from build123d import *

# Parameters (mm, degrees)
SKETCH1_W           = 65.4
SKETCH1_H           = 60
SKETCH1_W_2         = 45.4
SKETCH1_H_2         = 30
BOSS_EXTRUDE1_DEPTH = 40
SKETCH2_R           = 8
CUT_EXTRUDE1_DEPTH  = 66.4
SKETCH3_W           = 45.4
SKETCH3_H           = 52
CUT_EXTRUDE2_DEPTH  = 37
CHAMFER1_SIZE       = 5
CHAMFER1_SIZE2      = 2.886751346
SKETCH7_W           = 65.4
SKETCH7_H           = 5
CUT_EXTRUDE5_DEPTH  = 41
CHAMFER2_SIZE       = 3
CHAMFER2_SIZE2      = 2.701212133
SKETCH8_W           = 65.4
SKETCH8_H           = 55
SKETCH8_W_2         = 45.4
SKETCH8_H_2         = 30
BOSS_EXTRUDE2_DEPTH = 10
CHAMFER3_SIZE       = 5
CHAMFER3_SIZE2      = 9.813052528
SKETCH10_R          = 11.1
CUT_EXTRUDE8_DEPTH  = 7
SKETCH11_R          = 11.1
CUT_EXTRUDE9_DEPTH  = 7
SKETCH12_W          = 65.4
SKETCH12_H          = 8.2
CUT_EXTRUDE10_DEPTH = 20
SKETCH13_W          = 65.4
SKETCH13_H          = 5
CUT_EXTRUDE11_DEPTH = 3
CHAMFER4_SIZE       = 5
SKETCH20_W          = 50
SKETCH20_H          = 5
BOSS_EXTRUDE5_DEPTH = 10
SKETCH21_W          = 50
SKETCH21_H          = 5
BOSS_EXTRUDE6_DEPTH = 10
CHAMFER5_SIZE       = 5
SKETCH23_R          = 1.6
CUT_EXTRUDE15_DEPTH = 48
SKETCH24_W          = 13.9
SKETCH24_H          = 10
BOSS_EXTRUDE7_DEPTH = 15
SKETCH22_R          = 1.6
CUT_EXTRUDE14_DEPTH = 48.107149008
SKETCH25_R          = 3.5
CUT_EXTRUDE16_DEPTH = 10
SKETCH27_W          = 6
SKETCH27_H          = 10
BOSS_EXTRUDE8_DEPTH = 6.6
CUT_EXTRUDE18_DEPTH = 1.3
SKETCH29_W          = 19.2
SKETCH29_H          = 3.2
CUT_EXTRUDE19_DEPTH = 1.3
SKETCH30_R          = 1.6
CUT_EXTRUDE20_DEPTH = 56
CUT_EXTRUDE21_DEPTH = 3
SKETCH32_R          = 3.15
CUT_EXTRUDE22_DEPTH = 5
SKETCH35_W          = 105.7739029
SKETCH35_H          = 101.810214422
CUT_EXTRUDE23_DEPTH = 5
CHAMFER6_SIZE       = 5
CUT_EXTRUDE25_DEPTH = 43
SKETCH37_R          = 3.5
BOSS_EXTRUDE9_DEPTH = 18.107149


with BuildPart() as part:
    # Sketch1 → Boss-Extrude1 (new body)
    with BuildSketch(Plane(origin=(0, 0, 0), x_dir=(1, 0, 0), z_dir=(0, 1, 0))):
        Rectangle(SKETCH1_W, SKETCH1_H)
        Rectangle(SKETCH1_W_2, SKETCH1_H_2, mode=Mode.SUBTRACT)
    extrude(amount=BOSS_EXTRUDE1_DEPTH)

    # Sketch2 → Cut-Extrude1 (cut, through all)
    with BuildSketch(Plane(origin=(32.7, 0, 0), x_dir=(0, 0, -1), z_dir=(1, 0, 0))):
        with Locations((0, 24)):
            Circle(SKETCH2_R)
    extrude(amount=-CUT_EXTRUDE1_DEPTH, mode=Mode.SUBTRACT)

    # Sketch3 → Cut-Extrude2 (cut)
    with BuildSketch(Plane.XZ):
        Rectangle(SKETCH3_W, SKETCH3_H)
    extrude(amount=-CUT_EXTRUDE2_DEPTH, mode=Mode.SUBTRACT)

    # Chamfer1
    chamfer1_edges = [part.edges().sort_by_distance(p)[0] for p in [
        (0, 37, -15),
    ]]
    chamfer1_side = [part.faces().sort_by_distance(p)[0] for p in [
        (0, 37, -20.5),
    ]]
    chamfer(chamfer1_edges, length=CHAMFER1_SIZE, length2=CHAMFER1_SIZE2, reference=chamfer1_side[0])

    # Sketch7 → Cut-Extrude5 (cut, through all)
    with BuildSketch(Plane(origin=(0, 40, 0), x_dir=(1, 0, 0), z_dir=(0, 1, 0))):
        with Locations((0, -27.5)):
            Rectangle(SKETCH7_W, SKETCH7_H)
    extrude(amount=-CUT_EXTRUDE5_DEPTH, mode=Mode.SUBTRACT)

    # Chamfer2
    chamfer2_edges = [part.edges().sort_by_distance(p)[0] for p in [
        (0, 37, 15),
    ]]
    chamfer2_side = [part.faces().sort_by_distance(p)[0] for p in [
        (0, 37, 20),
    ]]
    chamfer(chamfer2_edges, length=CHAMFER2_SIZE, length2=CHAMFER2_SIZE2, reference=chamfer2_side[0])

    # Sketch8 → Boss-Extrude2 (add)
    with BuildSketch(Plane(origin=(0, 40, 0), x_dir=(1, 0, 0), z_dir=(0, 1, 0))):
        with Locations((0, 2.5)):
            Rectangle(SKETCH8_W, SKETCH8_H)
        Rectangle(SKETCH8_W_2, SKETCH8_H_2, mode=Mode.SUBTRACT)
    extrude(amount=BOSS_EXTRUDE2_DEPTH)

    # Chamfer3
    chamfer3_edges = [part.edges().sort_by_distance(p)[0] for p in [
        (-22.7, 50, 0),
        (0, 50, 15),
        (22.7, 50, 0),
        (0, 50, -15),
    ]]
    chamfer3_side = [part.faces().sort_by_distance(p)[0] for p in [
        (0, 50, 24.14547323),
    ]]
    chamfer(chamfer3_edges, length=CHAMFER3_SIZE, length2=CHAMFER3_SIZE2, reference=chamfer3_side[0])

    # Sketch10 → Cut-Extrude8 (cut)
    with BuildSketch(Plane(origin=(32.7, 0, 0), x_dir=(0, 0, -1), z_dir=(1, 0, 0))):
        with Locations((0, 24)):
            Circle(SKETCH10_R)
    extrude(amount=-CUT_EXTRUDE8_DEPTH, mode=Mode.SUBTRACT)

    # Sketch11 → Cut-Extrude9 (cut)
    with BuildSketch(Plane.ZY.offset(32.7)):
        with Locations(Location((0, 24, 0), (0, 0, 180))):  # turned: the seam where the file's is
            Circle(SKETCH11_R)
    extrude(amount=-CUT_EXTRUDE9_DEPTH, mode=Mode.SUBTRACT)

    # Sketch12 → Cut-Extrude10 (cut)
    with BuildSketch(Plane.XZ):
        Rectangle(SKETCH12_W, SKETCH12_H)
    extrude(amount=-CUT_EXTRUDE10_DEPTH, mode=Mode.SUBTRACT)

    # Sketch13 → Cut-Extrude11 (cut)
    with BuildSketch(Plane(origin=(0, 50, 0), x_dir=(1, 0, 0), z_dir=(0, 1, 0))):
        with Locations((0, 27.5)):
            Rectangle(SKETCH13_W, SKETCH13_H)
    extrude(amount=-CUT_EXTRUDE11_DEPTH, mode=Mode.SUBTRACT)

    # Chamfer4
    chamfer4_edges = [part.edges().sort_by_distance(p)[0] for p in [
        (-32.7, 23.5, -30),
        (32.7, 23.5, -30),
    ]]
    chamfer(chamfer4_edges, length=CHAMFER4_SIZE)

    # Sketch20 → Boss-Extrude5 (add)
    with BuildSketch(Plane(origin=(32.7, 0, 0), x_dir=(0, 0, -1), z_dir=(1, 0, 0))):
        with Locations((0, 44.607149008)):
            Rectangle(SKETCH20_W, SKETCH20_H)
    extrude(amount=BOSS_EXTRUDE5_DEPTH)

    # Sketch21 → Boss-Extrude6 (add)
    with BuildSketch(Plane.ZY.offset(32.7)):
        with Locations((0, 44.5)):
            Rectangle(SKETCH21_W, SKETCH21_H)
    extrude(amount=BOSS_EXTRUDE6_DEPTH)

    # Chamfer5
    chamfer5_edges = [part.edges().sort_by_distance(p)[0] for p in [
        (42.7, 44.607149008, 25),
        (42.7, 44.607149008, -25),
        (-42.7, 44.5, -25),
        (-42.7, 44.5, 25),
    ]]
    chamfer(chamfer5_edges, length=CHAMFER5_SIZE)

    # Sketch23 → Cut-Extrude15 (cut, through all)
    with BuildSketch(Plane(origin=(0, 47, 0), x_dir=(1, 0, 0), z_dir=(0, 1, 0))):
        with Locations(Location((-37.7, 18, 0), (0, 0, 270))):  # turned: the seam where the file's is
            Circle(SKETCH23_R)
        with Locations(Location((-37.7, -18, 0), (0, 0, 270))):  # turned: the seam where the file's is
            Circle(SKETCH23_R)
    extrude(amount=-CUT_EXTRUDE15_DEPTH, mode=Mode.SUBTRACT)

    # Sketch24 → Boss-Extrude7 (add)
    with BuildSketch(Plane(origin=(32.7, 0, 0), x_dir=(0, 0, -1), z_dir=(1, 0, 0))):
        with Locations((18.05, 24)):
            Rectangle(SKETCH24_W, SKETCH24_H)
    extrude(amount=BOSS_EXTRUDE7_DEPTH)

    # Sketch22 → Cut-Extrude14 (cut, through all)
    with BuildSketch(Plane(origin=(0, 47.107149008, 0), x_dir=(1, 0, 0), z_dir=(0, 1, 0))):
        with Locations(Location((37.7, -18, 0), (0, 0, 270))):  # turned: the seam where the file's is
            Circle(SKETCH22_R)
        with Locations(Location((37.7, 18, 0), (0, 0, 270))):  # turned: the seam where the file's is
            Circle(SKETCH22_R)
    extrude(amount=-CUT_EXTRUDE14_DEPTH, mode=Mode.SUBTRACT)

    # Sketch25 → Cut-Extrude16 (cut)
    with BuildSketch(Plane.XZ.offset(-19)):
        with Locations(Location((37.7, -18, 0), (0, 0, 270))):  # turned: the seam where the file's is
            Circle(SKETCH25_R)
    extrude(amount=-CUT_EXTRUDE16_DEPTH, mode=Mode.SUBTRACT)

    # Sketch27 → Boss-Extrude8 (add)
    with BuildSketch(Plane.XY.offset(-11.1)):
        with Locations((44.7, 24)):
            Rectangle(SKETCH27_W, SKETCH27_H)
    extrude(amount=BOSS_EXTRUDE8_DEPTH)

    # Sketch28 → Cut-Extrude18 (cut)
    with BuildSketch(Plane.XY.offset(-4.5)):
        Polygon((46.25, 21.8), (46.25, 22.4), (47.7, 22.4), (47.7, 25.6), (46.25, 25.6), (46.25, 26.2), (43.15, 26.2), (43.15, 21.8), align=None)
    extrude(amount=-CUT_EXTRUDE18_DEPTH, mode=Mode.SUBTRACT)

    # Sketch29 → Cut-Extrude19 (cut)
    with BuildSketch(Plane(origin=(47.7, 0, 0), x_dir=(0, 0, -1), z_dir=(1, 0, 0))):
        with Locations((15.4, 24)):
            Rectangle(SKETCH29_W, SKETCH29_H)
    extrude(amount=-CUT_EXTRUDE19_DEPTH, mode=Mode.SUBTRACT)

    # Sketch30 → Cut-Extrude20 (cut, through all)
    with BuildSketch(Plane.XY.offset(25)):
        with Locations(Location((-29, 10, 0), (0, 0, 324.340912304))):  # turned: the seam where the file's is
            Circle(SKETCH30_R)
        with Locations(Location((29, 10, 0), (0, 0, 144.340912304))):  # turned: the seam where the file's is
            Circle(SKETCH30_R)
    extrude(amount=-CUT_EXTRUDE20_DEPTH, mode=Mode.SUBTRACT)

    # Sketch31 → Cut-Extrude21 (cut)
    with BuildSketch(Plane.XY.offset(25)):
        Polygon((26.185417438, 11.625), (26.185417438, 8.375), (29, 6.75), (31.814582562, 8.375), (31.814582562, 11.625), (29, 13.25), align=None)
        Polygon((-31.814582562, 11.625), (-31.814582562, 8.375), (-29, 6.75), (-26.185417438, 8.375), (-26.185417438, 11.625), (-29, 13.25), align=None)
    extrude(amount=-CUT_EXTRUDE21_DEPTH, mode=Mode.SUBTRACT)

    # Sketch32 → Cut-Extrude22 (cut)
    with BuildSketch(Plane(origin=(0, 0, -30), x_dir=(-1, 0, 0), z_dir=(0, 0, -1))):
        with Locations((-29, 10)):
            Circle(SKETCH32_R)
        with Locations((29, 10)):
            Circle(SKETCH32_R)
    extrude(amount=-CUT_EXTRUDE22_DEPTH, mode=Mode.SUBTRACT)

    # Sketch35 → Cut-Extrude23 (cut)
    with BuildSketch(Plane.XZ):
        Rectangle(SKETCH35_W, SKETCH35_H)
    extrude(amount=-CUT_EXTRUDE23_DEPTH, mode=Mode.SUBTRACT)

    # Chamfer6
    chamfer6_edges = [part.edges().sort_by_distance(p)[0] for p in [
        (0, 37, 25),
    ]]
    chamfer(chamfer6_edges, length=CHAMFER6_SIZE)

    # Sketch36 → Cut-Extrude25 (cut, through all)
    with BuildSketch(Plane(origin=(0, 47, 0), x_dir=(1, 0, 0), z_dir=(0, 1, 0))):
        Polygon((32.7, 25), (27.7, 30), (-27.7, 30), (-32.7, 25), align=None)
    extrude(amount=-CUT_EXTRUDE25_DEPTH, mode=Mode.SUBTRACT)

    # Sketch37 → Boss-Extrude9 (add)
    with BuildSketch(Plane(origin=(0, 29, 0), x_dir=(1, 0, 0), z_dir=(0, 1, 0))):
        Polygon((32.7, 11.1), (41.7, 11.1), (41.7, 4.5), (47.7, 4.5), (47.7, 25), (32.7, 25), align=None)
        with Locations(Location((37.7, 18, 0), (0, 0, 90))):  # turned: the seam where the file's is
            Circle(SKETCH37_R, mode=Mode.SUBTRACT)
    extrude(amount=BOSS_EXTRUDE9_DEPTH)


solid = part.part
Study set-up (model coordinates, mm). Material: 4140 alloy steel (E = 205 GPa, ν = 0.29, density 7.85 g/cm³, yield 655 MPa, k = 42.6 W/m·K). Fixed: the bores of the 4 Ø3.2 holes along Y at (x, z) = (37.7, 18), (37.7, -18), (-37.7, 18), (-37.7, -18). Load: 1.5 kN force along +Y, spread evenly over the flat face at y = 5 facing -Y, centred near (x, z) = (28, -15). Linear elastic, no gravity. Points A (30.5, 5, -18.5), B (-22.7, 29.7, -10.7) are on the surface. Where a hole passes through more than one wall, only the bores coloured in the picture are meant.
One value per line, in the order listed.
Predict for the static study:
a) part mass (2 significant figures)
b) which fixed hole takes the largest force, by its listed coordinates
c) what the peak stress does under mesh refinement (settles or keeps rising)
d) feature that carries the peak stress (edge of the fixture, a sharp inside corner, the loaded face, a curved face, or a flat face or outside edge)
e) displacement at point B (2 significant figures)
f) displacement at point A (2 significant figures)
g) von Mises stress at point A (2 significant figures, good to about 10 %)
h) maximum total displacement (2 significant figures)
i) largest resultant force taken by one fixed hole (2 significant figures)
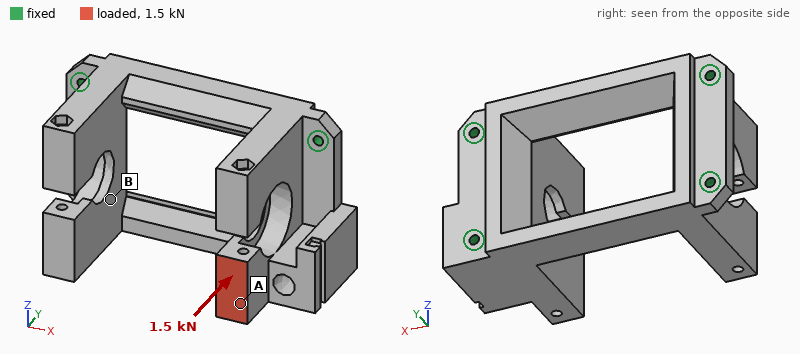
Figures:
410 g
(37.7, -18)
keeps rising
edge of the fixture
3.1 µm
14 µm
7.3 MPa
16 µm
1.2 kN
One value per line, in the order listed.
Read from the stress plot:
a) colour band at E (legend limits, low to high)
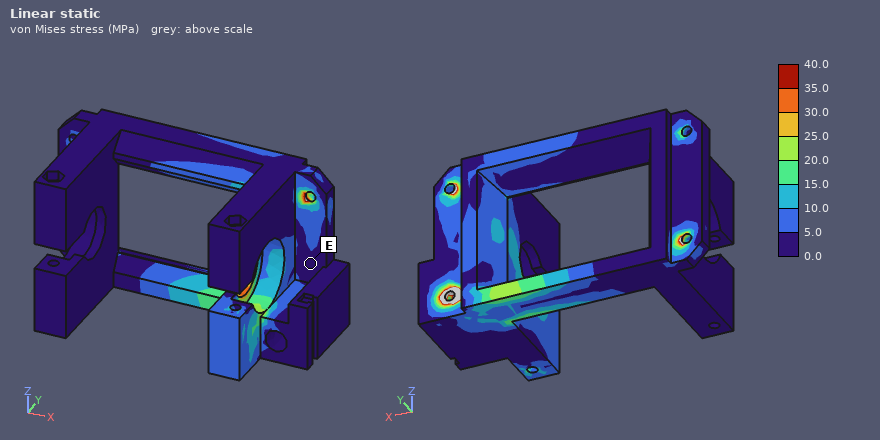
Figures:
0.0 to 5.0 MPa
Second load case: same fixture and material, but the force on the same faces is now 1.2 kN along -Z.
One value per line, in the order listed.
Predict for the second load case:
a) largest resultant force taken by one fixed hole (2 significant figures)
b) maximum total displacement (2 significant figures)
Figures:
1.3 kN
39 µm
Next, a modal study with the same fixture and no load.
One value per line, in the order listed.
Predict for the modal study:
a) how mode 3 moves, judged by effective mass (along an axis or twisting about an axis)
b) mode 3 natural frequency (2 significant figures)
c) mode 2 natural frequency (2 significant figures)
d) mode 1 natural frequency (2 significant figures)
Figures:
along X
4200 Hz
4000 Hz
2900 Hz
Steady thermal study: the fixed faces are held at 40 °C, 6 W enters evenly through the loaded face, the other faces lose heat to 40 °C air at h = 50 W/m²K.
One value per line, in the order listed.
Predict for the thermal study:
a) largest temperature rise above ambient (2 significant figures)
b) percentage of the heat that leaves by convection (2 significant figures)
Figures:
24 K
42 %
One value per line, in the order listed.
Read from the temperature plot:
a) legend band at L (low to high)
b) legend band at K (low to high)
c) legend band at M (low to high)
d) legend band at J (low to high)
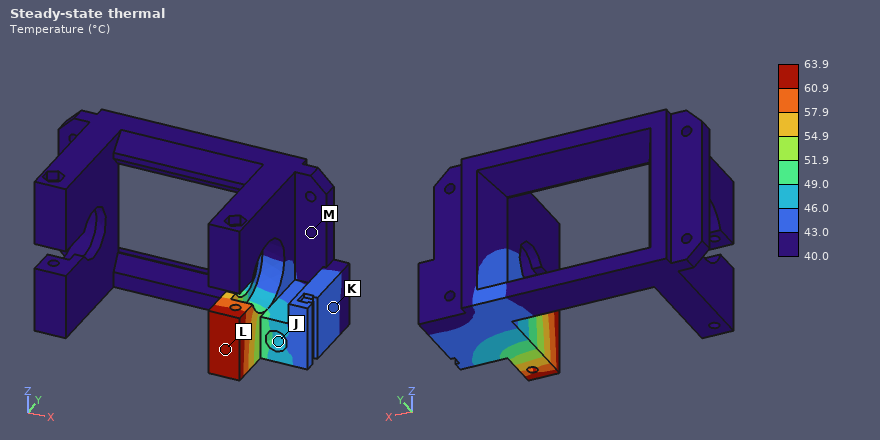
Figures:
60.9 to 63.9 °C
43.0 to 46.0 °C
40.0 to 43.0 °C
46.0 to 49.0 °C
